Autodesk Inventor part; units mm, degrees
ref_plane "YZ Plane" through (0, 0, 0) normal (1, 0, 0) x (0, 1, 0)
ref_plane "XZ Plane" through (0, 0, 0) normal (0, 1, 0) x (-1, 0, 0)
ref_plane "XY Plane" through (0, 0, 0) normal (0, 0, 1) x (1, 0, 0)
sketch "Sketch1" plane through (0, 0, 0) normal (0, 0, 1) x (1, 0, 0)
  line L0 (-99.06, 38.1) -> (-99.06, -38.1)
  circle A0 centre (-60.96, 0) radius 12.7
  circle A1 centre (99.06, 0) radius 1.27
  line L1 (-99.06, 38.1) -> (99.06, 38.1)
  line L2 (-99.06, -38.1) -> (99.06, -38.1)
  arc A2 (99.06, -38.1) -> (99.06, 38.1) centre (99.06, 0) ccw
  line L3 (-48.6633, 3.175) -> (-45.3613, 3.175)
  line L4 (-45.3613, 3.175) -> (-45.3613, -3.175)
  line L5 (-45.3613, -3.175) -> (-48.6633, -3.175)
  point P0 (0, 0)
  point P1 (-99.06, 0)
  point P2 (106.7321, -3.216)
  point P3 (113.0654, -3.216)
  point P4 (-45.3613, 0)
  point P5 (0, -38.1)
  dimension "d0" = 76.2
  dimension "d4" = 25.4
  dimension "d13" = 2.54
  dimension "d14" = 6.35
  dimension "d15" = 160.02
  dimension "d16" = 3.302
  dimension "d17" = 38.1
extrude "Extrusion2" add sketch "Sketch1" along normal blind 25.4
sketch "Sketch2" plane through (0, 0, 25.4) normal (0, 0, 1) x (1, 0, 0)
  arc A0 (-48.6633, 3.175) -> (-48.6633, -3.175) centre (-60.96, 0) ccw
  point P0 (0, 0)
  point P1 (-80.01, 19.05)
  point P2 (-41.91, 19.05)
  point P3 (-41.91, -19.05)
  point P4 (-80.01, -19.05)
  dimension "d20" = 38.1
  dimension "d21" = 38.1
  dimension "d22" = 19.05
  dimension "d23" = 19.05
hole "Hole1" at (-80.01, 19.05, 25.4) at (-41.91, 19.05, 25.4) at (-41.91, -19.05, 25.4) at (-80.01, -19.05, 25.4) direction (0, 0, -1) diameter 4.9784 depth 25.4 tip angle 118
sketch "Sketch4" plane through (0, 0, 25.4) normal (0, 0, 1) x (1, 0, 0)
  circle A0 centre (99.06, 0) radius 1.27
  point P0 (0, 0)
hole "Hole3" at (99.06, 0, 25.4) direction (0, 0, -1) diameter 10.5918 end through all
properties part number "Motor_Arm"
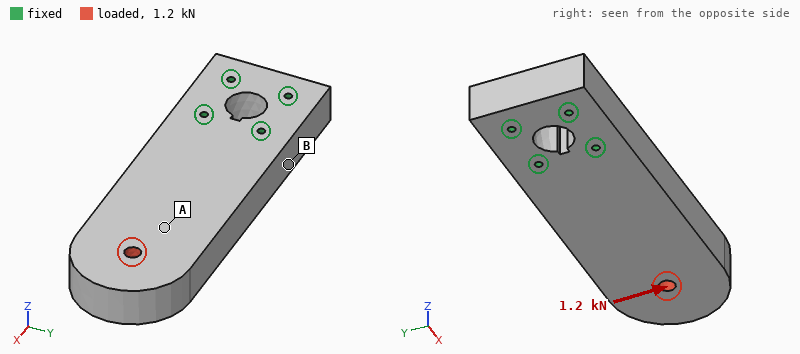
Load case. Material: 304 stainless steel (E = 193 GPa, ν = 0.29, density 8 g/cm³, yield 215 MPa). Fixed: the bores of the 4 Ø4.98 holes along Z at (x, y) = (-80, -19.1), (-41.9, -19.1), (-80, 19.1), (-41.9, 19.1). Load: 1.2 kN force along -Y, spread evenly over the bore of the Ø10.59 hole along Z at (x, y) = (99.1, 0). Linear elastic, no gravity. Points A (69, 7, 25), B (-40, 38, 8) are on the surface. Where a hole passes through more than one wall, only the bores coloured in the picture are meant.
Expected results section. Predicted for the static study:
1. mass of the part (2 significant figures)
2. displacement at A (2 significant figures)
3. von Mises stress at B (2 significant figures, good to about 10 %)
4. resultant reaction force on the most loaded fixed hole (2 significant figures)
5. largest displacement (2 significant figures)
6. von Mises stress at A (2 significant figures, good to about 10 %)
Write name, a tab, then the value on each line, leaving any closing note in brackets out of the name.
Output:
mass of the part	3.4 kg
displacement at A	6.7 µm
von Mises stress at B	5.3 MPa
resultant reaction force on the most loaded fixed hole	2.9 kN
largest displacement	12 µm
von Mises stress at A	1.6 MPa
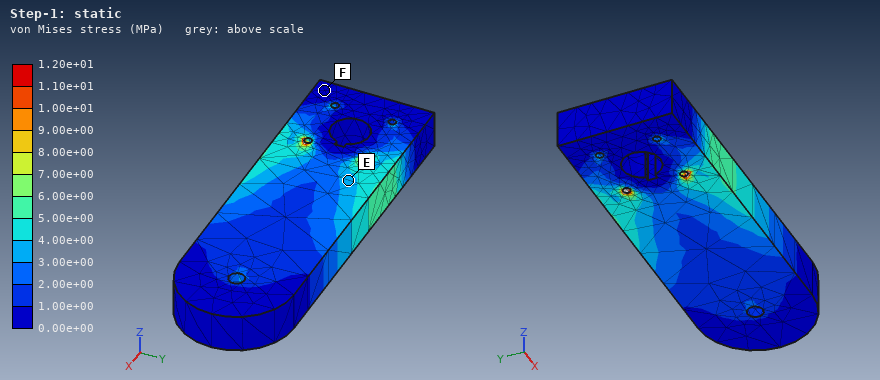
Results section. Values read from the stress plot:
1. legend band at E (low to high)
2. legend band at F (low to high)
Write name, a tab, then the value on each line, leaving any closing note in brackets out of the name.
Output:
legend band at E	3.00e+00 to 4.00e+00 MPa
legend band at F	0.00e+00 to 1.00e+00 MPa
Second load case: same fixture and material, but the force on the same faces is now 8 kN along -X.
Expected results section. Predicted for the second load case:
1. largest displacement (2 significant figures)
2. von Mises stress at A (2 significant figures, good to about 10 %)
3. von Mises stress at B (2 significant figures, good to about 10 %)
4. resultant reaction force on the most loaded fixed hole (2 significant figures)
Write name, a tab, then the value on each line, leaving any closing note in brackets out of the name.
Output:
largest displacement	4.1 µm
von Mises stress at A	5.6 MPa
von Mises stress at B	2.8 MPa
resultant reaction force on the most loaded fixed hole	3.5 kN
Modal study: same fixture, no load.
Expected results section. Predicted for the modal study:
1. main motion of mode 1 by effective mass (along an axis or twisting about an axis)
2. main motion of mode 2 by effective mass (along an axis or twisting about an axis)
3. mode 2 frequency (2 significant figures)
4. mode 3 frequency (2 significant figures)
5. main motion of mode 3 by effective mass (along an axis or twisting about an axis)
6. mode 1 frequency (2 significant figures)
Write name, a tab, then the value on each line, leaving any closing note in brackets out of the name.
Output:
main motion of mode 1 by effective mass	along Z
main motion of mode 2 by effective mass	along Y
mode 2 frequency	1600 Hz
mode 3 frequency	2800 Hz
main motion of mode 3 by effective mass	twisting about X
mode 1 frequency	640 Hz
